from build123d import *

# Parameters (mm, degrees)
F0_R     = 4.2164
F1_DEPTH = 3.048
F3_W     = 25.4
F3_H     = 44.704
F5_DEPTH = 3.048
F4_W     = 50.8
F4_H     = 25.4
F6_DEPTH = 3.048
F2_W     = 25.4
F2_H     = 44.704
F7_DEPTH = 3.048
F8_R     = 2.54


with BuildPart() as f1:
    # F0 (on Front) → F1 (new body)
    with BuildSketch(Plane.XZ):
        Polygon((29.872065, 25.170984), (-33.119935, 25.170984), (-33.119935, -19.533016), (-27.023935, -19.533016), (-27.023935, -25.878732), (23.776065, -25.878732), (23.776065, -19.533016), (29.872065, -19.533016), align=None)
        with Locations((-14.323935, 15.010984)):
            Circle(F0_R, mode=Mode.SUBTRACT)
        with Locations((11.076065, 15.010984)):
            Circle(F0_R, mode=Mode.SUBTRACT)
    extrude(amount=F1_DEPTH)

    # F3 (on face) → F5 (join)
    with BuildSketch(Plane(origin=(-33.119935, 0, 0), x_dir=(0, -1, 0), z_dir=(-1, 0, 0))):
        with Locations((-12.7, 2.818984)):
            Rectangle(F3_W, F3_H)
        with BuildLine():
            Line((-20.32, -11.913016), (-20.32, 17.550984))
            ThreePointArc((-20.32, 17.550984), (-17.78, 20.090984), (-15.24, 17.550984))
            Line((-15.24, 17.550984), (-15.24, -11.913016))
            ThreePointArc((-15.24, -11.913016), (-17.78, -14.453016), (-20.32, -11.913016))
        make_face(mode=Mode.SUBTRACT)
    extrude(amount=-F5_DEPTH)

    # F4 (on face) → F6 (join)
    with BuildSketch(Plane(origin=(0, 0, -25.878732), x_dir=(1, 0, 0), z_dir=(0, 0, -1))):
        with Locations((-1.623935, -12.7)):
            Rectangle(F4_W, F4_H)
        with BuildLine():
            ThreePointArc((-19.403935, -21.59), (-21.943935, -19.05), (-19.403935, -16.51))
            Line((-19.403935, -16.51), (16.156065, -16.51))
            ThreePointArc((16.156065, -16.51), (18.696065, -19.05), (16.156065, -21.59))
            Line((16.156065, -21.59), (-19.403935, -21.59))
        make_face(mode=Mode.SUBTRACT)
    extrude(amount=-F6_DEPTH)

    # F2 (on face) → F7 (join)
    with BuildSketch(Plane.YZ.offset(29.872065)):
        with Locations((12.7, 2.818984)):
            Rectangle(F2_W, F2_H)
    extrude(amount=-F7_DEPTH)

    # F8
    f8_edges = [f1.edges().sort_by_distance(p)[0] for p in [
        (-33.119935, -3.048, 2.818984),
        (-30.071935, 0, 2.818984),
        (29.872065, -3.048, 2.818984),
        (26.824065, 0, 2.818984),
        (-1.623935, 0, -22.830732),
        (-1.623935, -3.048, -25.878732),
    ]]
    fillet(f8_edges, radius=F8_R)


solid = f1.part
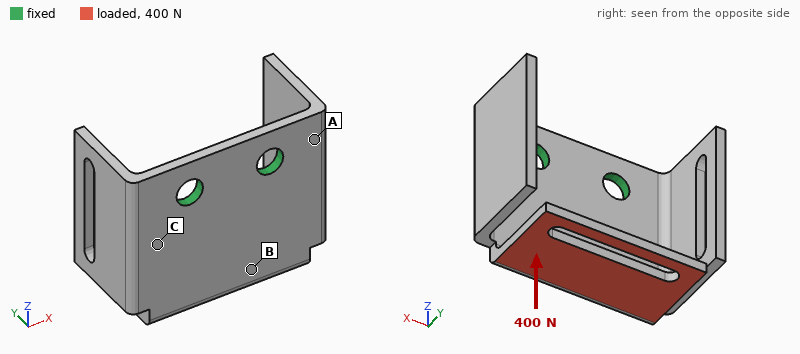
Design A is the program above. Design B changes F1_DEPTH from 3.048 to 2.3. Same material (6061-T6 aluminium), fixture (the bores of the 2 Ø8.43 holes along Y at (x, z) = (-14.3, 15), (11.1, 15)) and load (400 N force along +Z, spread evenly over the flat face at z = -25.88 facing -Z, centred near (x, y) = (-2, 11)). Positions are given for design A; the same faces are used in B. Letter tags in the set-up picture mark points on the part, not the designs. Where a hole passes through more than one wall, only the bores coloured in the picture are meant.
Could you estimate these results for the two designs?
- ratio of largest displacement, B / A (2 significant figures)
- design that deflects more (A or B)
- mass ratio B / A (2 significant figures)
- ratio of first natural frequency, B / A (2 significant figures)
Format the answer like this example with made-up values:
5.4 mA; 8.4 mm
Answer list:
1.8; B; 0.88; 0.72
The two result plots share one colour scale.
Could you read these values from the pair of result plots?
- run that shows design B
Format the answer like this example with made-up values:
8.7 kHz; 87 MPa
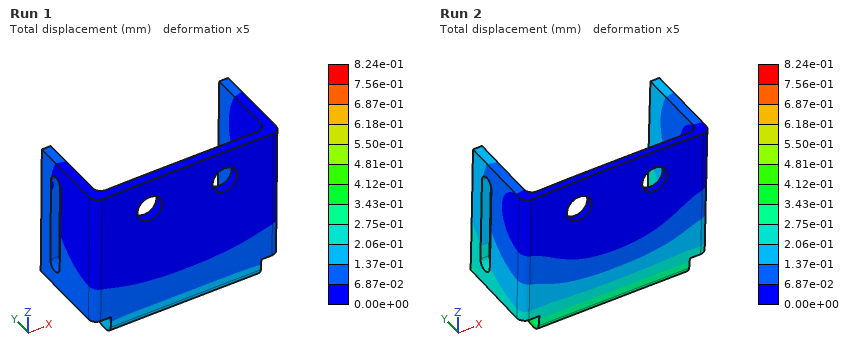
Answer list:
Run 2
